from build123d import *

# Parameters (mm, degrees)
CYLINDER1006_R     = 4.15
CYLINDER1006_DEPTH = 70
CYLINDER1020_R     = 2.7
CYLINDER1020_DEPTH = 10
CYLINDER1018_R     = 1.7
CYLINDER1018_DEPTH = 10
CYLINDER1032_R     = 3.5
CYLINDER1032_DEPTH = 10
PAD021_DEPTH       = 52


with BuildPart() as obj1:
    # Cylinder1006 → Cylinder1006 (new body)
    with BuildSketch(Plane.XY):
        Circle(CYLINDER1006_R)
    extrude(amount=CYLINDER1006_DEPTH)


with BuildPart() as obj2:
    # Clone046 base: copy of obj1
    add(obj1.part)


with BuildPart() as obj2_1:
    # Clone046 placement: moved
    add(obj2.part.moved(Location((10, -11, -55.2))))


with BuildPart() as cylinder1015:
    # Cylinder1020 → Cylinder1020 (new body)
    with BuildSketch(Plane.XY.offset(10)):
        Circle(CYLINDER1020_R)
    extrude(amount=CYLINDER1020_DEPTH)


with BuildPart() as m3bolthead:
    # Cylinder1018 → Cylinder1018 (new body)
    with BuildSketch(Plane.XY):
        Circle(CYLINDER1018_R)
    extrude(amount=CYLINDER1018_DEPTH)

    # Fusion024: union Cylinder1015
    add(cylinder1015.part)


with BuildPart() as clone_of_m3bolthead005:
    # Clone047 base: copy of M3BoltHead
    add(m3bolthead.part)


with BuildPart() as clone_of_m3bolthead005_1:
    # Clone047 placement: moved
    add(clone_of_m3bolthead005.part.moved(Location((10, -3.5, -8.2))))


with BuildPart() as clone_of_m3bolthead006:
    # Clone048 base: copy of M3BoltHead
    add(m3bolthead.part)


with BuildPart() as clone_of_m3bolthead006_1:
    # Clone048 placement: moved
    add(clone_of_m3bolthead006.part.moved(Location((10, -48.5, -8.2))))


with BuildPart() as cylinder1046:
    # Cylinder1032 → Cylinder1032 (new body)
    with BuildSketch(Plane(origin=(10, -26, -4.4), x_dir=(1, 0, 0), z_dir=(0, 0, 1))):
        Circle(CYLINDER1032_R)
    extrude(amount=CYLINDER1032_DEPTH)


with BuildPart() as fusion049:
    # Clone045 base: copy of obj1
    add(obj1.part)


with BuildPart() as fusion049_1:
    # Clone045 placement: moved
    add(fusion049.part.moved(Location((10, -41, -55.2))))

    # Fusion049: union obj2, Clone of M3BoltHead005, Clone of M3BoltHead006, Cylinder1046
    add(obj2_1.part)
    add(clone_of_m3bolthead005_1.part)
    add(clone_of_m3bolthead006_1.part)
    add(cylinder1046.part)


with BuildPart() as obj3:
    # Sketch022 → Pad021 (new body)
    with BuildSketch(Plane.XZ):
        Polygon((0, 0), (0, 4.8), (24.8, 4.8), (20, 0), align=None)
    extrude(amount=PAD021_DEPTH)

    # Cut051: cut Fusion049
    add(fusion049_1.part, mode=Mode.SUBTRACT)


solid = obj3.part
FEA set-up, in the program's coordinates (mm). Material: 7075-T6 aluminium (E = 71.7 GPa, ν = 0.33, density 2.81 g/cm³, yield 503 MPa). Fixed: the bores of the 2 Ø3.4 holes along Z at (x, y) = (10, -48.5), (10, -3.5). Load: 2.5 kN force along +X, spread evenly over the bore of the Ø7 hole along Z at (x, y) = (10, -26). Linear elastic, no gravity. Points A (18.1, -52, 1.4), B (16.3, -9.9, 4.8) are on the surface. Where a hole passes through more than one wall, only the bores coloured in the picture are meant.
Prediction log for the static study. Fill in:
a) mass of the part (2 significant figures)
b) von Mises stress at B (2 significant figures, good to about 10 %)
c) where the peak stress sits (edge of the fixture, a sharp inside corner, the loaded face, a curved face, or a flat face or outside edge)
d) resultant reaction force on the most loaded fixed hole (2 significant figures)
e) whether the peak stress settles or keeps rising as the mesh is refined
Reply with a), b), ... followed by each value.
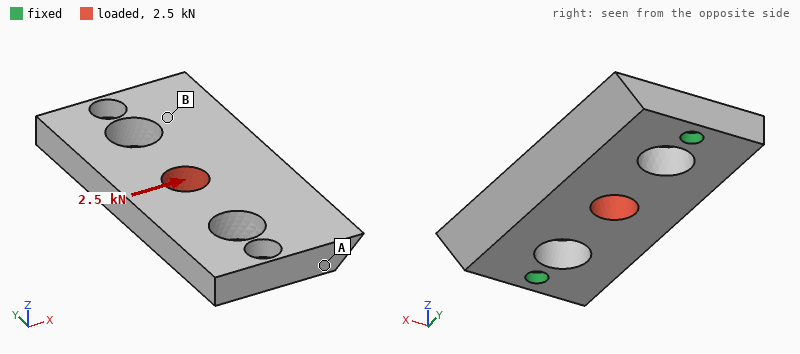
a) 13 g
b) 56 MPa
c) edge of the fixture
d) 1.3 kN
e) keeps rising
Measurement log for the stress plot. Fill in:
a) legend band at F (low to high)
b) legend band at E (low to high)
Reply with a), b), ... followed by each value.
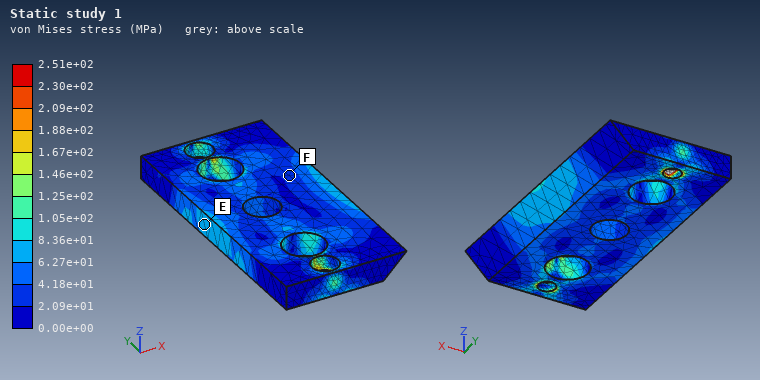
a) 2.09e+01 to 4.18e+01 MPa
b) 6.27e+01 to 8.36e+01 MPa
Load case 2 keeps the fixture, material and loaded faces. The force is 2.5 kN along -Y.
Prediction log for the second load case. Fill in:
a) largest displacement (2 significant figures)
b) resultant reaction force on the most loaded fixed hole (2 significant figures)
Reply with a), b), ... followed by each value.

a) 17 µm
b) 1.3 kN
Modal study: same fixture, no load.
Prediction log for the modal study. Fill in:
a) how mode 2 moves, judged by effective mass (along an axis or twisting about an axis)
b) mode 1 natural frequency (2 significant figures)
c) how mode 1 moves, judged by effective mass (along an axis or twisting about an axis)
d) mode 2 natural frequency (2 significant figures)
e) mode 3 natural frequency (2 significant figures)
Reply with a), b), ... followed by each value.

a) along Z
b) 5800 Hz
c) along Z
d) 7300 Hz
e) 14 kHz
